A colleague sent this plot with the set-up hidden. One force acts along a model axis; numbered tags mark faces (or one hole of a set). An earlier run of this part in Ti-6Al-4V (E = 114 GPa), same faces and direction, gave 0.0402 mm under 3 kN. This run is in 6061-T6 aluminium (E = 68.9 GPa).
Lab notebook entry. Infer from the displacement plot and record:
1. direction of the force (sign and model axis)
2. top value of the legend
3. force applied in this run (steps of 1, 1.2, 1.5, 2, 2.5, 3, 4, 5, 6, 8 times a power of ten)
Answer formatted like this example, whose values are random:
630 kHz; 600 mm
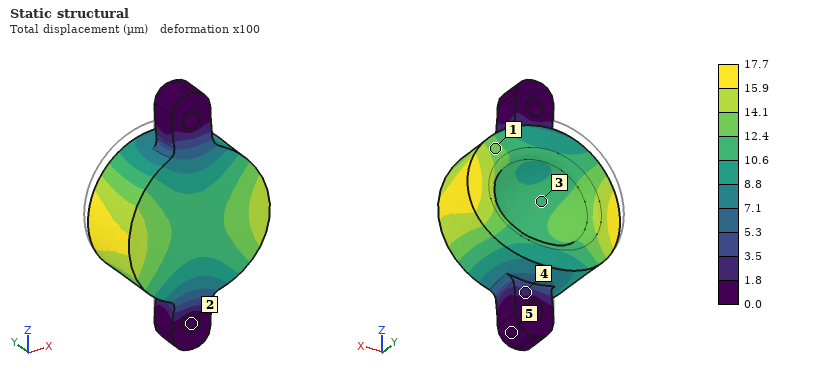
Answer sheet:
-Y; 17.7 µm; 800 N
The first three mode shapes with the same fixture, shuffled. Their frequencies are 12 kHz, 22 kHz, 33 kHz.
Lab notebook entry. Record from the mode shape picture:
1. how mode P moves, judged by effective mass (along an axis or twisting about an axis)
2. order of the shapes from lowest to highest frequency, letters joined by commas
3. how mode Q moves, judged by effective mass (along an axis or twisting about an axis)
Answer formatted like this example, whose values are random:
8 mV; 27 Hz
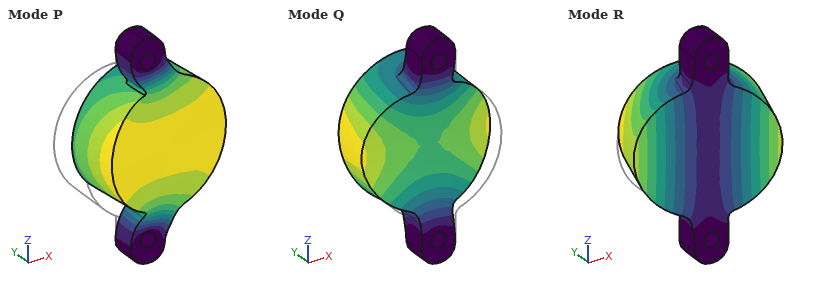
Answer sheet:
along X; R, Q, P; along Y
